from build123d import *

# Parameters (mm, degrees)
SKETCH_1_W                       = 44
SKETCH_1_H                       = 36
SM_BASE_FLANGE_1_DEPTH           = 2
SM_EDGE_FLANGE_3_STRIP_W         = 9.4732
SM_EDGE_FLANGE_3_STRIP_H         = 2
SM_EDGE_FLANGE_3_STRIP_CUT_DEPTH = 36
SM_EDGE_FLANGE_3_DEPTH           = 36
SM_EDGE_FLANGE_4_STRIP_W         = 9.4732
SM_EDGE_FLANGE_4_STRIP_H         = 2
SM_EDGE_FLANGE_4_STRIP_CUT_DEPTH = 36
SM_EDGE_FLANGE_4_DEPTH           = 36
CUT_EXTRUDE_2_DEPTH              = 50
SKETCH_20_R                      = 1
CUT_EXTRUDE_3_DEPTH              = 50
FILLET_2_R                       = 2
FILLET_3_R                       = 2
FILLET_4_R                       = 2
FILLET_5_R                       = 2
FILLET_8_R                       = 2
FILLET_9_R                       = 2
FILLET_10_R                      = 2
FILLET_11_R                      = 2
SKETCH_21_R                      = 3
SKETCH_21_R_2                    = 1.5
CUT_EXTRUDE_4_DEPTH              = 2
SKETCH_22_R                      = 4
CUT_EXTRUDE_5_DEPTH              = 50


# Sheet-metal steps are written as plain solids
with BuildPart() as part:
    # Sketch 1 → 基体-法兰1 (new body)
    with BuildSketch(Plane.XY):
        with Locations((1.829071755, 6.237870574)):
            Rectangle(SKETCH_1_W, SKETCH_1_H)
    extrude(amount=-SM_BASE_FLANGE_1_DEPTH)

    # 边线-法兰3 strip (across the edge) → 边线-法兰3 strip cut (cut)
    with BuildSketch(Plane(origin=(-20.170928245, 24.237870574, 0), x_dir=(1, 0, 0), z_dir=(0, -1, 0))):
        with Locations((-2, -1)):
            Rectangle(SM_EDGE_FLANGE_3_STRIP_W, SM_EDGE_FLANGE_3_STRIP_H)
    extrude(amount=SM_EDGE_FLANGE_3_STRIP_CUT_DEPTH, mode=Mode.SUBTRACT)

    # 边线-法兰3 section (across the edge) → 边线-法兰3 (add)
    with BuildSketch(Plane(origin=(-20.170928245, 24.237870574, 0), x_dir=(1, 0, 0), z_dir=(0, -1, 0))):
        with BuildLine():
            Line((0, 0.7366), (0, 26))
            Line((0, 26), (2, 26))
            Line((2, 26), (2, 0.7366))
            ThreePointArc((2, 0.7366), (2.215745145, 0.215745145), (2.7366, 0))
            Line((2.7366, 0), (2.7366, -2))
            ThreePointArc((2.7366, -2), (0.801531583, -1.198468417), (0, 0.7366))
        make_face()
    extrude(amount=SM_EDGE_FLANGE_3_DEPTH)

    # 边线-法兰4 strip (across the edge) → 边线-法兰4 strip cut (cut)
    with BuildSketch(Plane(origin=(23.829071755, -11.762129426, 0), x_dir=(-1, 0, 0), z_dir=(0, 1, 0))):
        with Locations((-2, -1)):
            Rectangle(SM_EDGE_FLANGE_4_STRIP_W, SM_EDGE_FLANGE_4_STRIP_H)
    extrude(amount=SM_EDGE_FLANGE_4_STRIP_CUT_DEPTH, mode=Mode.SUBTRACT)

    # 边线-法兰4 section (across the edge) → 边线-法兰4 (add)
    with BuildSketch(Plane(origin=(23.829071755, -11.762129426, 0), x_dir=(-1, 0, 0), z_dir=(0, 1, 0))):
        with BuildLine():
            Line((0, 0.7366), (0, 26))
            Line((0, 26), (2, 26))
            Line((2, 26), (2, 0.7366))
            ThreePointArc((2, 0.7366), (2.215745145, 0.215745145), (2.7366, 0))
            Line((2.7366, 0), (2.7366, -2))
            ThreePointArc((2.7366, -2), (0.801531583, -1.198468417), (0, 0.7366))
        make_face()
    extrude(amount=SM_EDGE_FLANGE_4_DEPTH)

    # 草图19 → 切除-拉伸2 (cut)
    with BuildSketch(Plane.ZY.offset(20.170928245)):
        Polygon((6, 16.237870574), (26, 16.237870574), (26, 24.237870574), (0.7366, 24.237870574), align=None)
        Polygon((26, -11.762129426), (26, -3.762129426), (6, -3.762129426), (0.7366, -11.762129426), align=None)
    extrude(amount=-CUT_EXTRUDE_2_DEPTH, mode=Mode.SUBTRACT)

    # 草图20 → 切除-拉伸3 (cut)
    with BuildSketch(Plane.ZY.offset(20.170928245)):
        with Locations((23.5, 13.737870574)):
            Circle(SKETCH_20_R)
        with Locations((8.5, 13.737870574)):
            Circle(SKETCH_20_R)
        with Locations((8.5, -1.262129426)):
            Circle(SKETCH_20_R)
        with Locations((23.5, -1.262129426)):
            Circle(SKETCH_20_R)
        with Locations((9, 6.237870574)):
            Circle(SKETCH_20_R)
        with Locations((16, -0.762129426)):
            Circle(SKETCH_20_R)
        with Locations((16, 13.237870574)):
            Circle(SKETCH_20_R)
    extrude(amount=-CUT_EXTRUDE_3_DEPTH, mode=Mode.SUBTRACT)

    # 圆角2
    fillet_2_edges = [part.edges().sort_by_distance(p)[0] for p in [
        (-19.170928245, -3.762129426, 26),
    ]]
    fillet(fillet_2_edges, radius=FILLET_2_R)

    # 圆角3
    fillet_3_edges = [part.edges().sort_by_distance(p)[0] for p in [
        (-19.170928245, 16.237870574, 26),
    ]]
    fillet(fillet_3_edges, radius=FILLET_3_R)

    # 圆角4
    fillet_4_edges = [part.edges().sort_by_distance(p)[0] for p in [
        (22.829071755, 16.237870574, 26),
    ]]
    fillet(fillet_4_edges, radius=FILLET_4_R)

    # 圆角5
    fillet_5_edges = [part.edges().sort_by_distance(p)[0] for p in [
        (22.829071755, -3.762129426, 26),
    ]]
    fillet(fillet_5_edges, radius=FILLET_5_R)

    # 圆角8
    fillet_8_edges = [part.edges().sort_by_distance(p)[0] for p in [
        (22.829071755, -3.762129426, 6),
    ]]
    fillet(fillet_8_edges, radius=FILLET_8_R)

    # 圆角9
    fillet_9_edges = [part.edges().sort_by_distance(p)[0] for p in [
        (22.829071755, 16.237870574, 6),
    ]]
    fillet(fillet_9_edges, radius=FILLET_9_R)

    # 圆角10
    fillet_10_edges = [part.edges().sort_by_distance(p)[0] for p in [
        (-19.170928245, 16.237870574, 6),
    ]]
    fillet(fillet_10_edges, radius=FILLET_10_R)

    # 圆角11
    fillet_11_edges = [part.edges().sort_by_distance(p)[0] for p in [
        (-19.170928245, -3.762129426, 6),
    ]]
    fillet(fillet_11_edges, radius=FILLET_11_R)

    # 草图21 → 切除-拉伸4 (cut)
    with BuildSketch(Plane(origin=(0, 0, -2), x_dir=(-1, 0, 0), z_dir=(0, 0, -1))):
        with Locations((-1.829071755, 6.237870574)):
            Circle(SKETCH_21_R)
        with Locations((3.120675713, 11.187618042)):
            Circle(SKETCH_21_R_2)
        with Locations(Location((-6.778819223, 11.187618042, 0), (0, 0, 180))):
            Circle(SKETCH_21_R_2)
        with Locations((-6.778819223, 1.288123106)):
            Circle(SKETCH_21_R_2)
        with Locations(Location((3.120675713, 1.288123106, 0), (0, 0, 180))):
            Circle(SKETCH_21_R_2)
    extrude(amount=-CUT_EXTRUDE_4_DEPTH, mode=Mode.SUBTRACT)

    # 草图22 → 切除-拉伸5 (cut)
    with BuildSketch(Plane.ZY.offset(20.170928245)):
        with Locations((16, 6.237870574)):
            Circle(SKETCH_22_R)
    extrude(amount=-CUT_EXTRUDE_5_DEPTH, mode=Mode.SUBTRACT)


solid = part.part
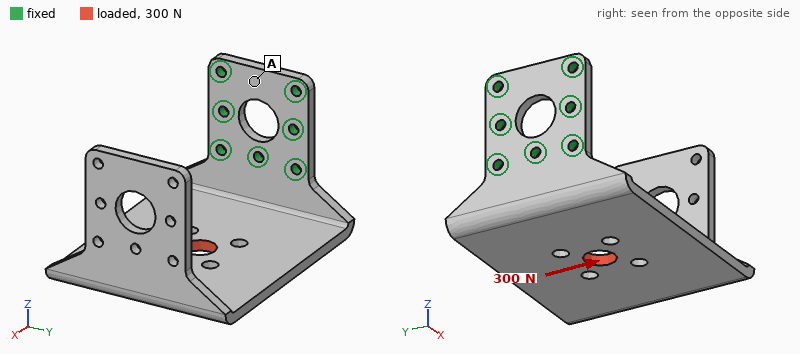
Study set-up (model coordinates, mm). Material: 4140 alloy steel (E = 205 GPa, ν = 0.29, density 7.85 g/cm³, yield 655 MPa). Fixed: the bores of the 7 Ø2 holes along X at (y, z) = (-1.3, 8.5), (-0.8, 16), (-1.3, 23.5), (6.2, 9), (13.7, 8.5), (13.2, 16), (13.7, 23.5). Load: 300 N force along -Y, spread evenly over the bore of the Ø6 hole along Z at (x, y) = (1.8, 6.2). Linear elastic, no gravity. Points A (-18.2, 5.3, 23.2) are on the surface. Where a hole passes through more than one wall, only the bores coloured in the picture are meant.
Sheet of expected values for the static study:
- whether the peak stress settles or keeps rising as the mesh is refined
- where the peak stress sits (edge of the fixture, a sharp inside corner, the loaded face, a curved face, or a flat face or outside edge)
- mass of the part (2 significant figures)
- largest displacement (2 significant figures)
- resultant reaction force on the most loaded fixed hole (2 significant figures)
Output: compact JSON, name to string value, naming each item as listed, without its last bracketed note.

{"whether the peak stress settles or keeps rising as the mesh is refined": "keeps rising", "where the peak stress sits": "edge of the fixture", "mass of the part": "39 g", "largest displacement": "0.25 mm", "resultant reaction force on the most loaded fixed hole": "440 N"}
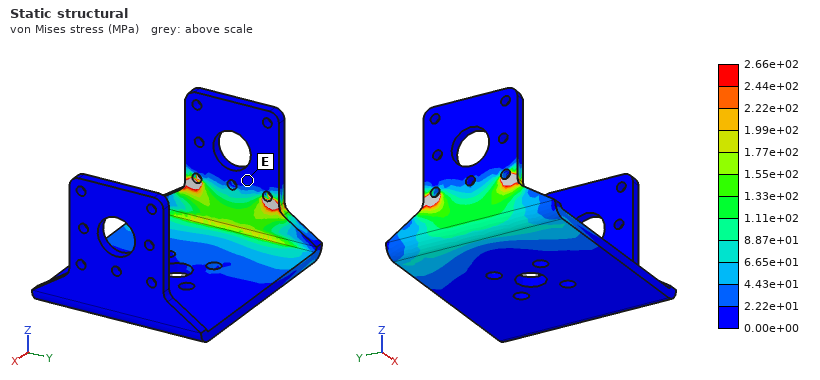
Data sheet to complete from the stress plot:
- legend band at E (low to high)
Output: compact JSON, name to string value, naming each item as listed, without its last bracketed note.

{"legend band at E": "0.00e+00 to 2.22e+01 MPa"}
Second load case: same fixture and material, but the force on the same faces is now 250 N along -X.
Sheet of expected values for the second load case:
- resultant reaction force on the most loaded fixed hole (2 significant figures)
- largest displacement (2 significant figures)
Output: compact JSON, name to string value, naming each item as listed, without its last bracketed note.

{"resultant reaction force on the most loaded fixed hole": "110 N", "largest displacement": "0.17 mm"}
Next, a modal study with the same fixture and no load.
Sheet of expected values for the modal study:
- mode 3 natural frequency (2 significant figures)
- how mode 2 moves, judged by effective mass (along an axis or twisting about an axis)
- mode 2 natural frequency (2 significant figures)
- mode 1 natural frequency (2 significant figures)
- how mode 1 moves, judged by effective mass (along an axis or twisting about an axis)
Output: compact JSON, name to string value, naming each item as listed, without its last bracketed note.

{"mode 3 natural frequency": "1600 Hz", "how mode 2 moves, judged by effective mass": "along Y", "mode 2 natural frequency": "900 Hz", "mode 1 natural frequency": "410 Hz", "how mode 1 moves, judged by effective mass": "along Z"}
